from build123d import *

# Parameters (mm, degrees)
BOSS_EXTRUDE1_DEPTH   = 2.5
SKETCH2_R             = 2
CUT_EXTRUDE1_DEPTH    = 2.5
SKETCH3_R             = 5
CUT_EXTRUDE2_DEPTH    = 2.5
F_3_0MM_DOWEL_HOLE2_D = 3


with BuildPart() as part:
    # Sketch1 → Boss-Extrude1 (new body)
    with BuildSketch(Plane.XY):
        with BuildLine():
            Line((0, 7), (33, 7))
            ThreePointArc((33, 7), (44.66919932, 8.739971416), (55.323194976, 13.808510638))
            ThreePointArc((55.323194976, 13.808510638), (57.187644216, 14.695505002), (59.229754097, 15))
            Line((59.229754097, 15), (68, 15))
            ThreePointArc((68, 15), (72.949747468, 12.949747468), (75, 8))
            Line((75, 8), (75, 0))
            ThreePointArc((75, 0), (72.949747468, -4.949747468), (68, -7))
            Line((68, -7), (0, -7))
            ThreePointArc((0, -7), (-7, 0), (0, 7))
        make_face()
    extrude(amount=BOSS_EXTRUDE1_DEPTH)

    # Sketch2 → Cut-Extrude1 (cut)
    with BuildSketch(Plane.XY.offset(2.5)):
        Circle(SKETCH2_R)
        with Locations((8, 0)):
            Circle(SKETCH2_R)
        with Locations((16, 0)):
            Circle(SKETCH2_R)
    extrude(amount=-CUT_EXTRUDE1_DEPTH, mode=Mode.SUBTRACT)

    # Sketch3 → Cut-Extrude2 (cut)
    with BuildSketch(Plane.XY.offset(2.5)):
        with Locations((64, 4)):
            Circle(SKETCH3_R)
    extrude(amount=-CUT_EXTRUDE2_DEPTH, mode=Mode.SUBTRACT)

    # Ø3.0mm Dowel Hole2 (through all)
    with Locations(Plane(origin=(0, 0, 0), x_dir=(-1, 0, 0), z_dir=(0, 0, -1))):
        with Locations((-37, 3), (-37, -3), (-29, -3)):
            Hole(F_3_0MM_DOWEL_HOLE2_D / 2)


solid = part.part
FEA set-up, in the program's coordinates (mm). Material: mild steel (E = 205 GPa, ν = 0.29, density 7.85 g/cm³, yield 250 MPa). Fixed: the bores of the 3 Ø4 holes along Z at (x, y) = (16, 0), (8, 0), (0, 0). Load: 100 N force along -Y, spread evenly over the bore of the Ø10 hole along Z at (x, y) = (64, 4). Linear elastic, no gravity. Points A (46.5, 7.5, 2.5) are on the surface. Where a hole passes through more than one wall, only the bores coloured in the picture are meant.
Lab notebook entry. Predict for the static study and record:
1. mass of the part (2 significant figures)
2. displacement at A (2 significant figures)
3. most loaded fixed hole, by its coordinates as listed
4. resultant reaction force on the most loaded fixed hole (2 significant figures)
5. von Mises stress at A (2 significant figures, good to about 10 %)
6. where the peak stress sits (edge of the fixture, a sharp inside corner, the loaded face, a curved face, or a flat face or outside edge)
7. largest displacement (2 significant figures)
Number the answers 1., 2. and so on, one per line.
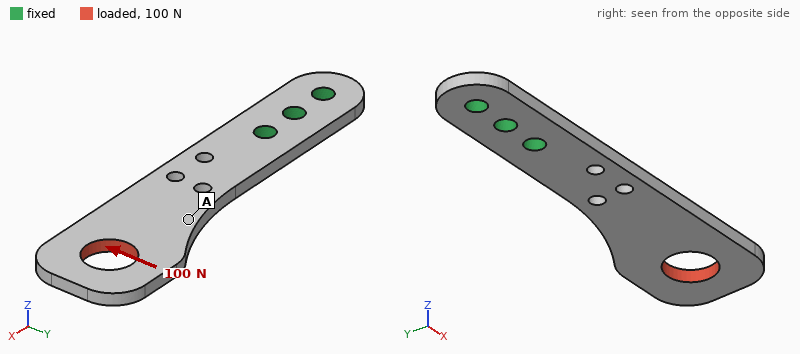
1. 23 g
2. 24 µm
3. (16, 0)
4. 340 N
5. 12 MPa
6. edge of the fixture
7. 56 µm
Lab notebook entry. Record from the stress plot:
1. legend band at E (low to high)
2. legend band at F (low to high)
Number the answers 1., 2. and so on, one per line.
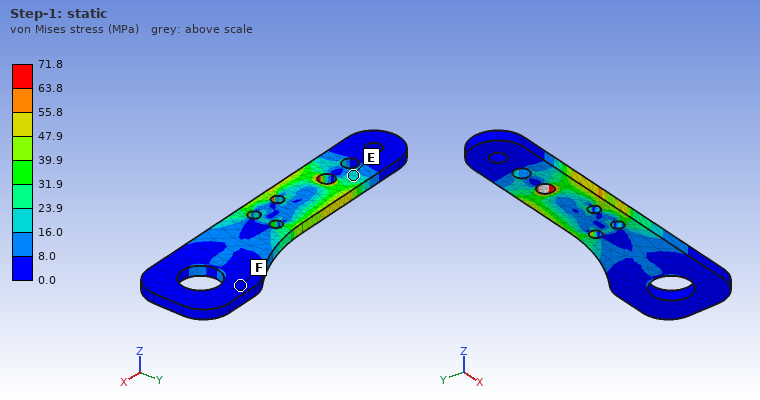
1. 16.0 to 23.9 MPa
2. 0.0 to 8.0 MPa
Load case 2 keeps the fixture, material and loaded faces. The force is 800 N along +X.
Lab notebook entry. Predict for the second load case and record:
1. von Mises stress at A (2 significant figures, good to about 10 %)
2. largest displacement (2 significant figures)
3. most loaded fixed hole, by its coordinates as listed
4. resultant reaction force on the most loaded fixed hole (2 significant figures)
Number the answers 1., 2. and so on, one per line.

1. 37 MPa
2. 47 µm
3. (16, 0)
4. 680 N
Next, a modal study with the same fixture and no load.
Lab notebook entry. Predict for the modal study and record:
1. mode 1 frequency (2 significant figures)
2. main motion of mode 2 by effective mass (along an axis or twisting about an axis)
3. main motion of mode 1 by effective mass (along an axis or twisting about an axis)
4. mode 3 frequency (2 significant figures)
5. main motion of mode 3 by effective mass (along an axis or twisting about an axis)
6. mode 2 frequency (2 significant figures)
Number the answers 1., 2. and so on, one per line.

1. 540 Hz
2. along Y
3. along Z
4. 2800 Hz
5. twisting about X
6. 2500 Hz
